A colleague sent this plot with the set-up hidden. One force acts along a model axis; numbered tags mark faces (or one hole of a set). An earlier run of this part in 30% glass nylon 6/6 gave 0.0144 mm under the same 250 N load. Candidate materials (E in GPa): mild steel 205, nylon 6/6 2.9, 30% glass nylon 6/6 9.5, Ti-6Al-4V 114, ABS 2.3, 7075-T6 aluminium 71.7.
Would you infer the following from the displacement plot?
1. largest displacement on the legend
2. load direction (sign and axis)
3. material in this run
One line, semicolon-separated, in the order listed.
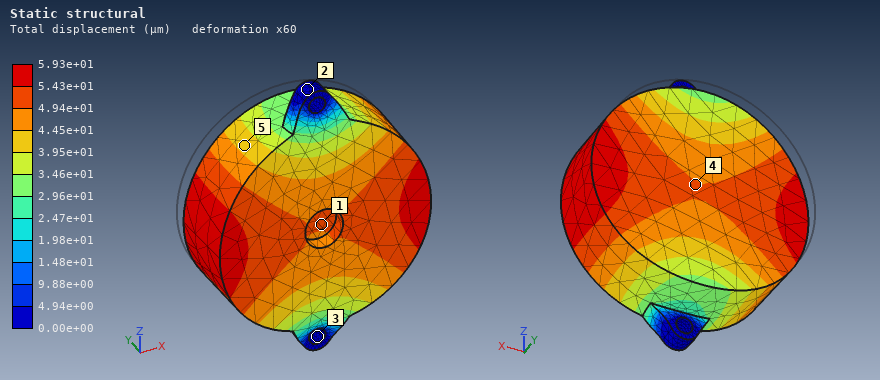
5.93e+01 µm; -Y; ABS
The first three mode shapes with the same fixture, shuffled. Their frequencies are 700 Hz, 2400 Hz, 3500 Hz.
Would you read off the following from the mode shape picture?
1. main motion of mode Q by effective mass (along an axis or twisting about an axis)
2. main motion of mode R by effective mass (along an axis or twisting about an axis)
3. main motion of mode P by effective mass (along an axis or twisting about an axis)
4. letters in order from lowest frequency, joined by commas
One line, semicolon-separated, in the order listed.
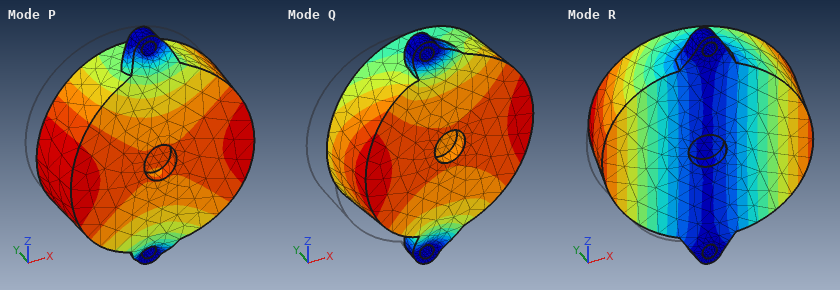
along X; along X; along Y; R, P, Q
